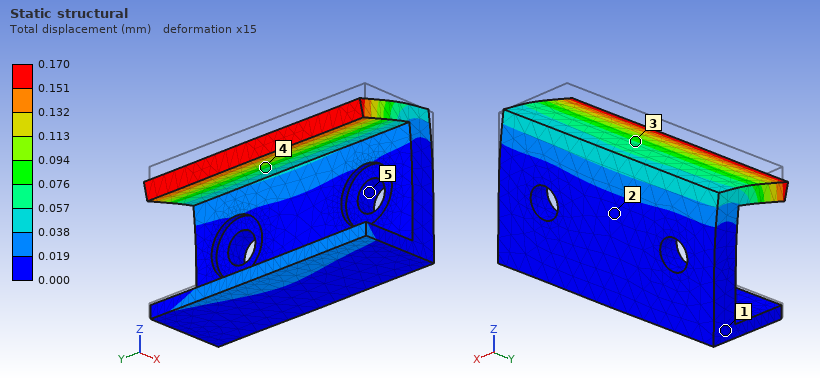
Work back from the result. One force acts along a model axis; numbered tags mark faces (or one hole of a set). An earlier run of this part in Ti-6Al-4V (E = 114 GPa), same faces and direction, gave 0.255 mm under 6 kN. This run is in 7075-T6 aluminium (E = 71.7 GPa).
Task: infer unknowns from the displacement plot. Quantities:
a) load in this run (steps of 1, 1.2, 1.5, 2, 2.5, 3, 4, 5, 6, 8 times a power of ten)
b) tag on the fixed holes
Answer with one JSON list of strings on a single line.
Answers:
["2.5 kN", "5"]
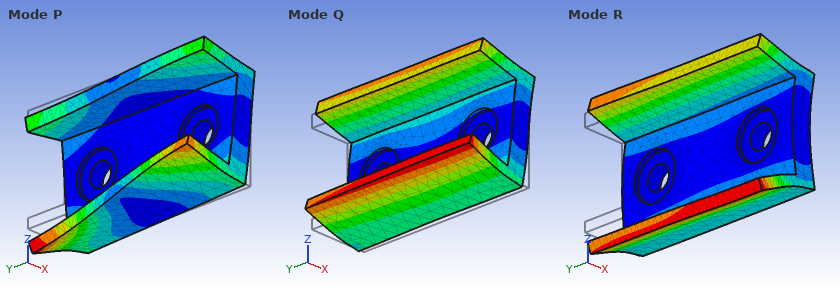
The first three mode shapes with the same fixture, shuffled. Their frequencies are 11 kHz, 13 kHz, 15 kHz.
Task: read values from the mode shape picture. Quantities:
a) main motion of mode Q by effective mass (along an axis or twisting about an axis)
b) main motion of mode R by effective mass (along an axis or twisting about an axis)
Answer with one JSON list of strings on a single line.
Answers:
["along Z", "along X"]
